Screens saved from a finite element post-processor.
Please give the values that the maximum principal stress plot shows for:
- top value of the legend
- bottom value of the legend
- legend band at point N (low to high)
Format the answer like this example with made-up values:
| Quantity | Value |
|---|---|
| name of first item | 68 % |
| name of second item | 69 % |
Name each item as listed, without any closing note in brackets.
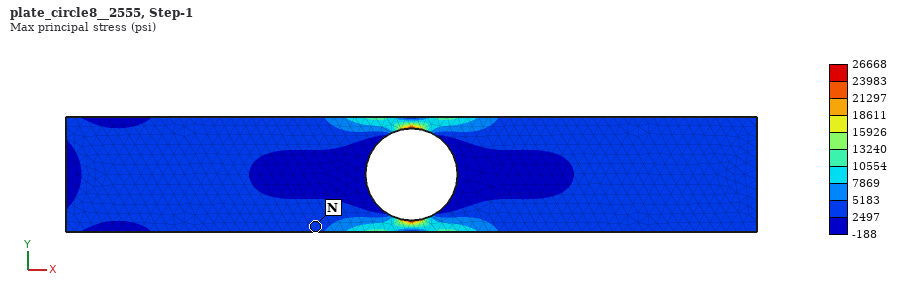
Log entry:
| Quantity | Value |
|---|---|
| top value of the legend | 26668 psi |
| bottom value of the legend | -188 psi |
| legend band at point N | 2497 to 5183 psi |
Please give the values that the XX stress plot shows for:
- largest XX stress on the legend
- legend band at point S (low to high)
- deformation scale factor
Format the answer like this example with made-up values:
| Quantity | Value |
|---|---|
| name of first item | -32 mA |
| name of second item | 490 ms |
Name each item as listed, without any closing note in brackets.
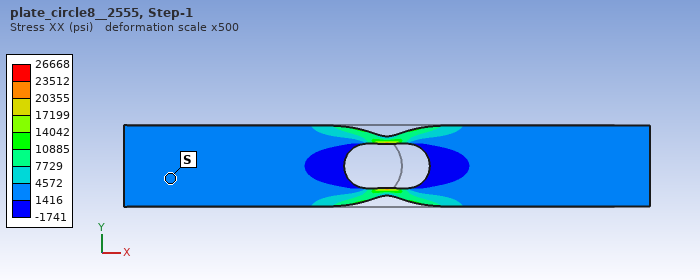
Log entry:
| Quantity | Value |
|---|---|
| largest XX stress on the legend | 26668 psi |
| legend band at point S | 1416 to 4572 psi |
| deformation scale factor | 500 |
